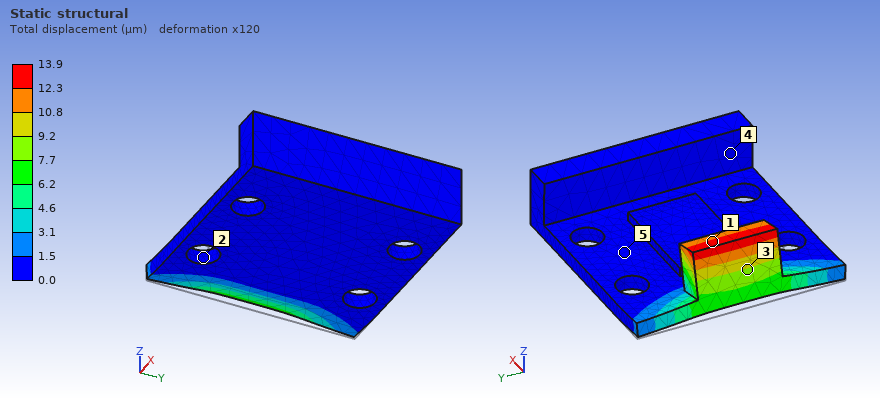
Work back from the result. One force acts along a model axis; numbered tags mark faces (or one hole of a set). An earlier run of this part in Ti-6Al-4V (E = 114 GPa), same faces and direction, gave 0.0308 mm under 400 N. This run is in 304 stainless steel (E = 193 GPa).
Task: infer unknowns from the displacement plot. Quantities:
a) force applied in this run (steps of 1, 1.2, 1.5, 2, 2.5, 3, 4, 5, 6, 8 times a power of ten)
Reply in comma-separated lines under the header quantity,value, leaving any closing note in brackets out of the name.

quantity,value
force applied in this run,300 N
